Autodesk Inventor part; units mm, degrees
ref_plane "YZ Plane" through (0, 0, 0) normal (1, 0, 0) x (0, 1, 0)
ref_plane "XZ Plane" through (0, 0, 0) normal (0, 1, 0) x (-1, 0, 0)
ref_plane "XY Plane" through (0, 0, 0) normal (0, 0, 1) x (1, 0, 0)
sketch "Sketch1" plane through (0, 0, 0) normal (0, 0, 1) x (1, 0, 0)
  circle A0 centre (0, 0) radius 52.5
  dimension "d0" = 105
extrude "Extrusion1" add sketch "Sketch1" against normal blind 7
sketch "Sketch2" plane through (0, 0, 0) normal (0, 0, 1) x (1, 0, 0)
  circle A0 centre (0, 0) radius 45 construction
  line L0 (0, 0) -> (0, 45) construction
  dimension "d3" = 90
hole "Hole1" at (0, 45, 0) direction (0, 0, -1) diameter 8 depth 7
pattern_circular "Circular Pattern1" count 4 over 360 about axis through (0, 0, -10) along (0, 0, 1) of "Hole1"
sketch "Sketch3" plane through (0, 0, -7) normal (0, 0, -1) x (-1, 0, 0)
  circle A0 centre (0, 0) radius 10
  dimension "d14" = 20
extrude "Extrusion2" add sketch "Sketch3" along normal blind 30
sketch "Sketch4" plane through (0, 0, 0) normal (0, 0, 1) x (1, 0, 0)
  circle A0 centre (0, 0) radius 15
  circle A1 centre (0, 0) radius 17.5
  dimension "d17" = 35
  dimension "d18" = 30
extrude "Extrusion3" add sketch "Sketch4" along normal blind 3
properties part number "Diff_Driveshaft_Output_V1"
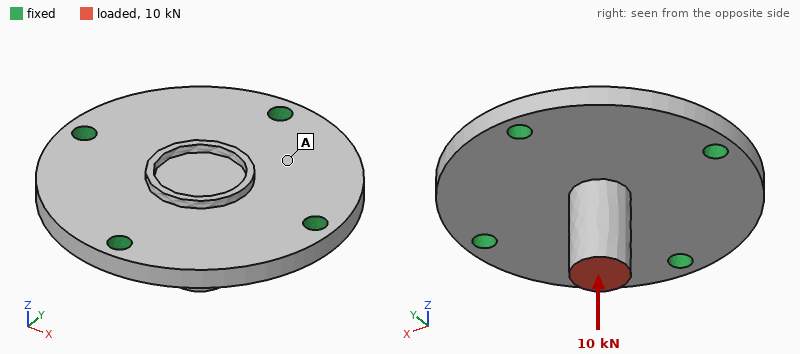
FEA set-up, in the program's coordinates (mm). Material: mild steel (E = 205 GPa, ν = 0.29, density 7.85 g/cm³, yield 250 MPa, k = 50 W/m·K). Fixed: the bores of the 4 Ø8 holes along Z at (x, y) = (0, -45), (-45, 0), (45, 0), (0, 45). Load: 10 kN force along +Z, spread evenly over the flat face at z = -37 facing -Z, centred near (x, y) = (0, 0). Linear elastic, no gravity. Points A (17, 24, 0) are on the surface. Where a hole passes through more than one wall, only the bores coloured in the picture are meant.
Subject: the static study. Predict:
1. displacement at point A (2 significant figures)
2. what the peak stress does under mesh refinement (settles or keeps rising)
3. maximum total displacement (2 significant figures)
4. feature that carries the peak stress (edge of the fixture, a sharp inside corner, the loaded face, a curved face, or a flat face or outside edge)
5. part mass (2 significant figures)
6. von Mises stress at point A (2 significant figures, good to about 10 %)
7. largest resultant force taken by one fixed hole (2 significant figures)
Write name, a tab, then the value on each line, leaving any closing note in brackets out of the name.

displacement at point A	22 µm
what the peak stress does under mesh refinement	keeps rising
maximum total displacement	58 µm
feature that carries the peak stress	edge of the fixture
part mass	540 g
von Mises stress at point A	54 MPa
largest resultant force taken by one fixed hole	2.5 kN
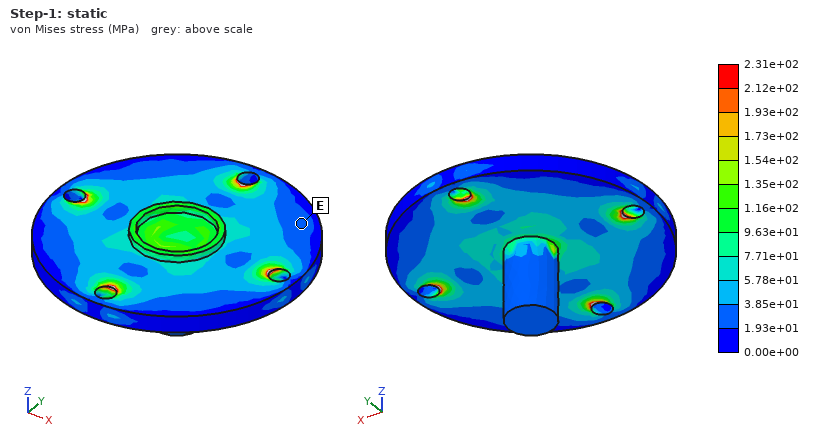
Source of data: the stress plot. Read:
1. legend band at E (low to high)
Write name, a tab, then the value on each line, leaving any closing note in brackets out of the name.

legend band at E	1.93e+01 to 3.85e+01 MPa
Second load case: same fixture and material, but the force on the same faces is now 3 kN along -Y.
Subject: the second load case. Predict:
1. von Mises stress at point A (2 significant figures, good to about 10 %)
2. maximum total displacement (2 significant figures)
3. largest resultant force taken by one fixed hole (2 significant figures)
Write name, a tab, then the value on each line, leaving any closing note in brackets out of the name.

von Mises stress at point A	24 MPa
maximum total displacement	70 µm
largest resultant force taken by one fixed hole	1.7 kN
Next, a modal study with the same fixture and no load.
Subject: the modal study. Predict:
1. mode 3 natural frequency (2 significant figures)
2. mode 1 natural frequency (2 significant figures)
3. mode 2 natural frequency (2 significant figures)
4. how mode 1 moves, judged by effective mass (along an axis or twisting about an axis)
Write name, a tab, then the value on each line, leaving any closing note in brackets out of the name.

mode 3 natural frequency	6100 Hz
mode 1 natural frequency	5300 Hz
mode 2 natural frequency	6100 Hz
how mode 1 moves, judged by effective mass	along Z
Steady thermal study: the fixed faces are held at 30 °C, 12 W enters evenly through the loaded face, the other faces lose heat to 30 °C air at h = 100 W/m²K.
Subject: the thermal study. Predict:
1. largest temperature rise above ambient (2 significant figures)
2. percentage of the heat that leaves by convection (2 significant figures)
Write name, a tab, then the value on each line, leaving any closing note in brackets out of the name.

largest temperature rise above ambient	27 K
percentage of the heat that leaves by convection	55 %
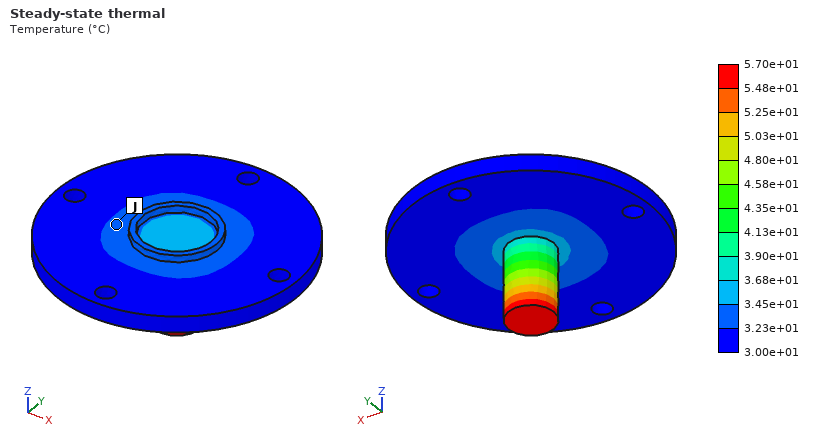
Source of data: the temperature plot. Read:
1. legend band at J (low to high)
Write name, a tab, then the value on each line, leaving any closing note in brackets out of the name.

legend band at J	3.23e+01 to 3.45e+01 °C
